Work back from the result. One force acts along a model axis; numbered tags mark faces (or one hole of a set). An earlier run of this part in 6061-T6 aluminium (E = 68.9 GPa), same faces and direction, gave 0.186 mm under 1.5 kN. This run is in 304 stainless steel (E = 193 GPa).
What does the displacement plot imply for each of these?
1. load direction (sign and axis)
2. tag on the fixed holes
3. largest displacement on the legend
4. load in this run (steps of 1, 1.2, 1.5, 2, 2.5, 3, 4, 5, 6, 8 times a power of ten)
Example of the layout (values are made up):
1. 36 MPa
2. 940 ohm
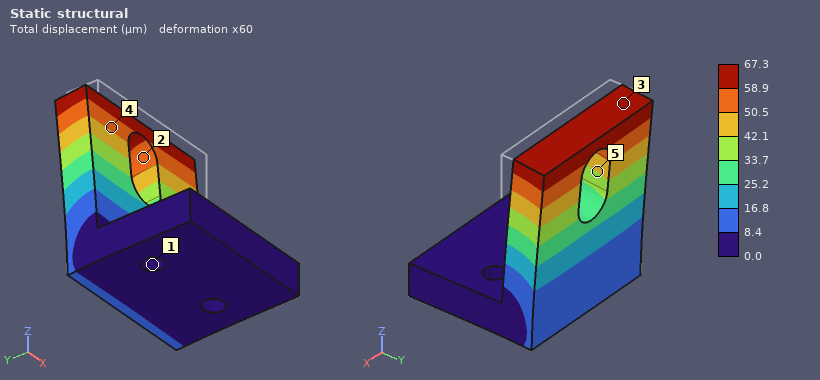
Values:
1. +Y
2. 1
3. 67.3 µm
4. 1.5 kN
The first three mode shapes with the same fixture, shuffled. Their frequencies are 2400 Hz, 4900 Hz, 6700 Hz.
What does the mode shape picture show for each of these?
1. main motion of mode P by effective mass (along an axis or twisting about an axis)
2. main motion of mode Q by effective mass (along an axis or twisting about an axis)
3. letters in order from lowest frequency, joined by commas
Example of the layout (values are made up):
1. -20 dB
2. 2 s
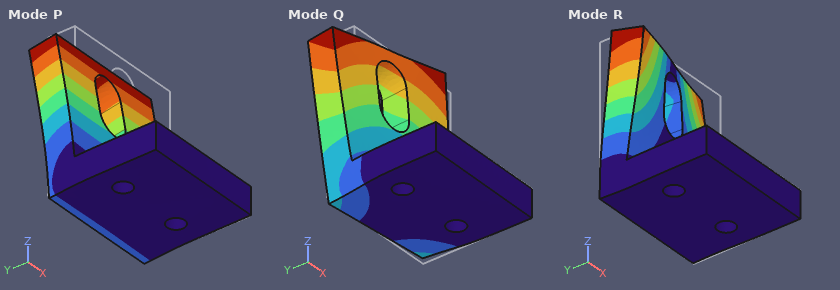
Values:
1. along Y
2. along X
3. P, Q, R
